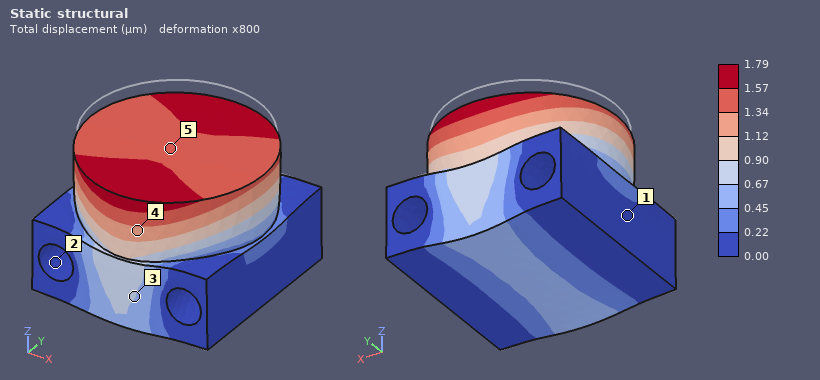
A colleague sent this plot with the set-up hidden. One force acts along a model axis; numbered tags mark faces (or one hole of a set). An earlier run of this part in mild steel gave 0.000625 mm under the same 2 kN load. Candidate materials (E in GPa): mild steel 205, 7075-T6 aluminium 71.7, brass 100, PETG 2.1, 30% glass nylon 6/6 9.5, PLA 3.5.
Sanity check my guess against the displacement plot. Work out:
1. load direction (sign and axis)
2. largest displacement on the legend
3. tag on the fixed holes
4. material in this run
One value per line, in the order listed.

-Z
1.79 µm
2
7075-T6 aluminium
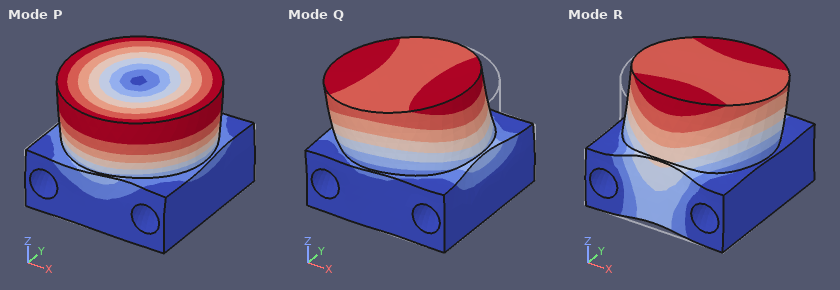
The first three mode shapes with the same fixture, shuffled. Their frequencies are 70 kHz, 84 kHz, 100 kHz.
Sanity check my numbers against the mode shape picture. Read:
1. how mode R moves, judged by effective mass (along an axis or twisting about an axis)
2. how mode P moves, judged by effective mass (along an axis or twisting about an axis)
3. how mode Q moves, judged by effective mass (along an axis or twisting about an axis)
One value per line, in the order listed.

along Y
twisting about Z
along X
